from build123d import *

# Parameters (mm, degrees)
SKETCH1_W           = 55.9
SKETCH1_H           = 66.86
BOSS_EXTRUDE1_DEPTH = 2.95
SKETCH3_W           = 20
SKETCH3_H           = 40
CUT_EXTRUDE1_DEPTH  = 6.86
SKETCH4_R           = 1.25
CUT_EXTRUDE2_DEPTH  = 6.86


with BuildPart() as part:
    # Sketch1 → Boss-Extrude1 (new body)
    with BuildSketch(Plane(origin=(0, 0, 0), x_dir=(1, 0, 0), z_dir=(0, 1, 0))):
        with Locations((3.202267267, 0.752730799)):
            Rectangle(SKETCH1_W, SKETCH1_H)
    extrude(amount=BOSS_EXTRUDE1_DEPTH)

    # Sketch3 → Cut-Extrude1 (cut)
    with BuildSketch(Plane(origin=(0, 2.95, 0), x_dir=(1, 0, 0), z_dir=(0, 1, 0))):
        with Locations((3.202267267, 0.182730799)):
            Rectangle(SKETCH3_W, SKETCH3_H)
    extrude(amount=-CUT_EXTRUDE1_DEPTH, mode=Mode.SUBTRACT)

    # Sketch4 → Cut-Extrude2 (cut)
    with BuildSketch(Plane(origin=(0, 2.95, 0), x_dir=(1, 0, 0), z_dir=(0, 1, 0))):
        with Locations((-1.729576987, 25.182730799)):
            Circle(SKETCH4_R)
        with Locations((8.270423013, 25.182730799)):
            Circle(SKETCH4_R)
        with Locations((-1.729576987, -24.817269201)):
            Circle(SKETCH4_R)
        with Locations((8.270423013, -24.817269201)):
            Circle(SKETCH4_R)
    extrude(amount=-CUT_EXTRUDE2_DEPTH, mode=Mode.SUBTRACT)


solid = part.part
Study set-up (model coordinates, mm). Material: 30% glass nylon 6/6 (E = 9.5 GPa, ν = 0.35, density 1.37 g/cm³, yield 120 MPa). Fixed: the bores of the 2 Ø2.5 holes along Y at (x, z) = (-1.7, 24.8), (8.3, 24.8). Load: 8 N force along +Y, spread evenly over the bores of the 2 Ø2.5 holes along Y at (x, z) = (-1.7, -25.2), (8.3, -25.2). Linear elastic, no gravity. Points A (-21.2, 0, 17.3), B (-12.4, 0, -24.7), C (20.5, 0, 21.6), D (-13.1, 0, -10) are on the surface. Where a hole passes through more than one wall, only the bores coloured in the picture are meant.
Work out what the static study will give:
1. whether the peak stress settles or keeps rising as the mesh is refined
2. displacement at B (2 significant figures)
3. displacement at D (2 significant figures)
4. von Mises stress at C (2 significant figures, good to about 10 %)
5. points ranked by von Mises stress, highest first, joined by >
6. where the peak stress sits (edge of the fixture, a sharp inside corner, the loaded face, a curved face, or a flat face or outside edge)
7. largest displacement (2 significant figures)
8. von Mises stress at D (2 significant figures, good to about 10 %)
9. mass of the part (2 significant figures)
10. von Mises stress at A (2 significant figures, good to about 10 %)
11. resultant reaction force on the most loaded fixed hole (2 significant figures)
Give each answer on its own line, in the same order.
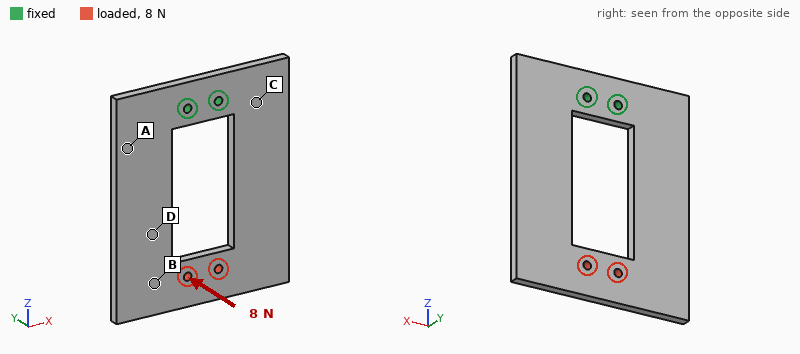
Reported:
keeps rising
0.69 mm
0.43 mm
6.5 MPa
C > A > D > B
edge of the fixture
0.88 mm
2.6 MPa
12 g
5.1 MPa
4.0 N
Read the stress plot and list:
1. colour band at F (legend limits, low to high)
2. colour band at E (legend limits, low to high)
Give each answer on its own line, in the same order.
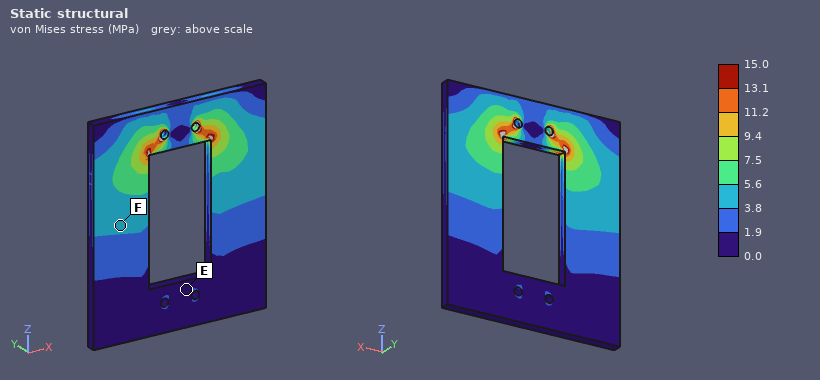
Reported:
3.8 to 5.6 MPa
0.0 to 1.9 MPa
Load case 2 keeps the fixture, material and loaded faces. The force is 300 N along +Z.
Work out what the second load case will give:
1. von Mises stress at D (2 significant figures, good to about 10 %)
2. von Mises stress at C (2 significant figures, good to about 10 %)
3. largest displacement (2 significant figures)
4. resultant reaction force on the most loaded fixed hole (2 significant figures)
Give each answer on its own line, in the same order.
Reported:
4.6 MPa
2.9 MPa
78 µm
160 N
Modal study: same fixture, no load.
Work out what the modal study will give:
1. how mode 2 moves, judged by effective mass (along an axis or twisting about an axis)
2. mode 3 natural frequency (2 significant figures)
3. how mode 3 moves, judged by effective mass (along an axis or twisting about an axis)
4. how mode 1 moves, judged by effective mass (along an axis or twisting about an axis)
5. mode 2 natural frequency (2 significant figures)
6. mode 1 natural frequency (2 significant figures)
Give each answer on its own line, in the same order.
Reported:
twisting about Z
1000 Hz
along X
along Y
540 Hz
240 Hz
